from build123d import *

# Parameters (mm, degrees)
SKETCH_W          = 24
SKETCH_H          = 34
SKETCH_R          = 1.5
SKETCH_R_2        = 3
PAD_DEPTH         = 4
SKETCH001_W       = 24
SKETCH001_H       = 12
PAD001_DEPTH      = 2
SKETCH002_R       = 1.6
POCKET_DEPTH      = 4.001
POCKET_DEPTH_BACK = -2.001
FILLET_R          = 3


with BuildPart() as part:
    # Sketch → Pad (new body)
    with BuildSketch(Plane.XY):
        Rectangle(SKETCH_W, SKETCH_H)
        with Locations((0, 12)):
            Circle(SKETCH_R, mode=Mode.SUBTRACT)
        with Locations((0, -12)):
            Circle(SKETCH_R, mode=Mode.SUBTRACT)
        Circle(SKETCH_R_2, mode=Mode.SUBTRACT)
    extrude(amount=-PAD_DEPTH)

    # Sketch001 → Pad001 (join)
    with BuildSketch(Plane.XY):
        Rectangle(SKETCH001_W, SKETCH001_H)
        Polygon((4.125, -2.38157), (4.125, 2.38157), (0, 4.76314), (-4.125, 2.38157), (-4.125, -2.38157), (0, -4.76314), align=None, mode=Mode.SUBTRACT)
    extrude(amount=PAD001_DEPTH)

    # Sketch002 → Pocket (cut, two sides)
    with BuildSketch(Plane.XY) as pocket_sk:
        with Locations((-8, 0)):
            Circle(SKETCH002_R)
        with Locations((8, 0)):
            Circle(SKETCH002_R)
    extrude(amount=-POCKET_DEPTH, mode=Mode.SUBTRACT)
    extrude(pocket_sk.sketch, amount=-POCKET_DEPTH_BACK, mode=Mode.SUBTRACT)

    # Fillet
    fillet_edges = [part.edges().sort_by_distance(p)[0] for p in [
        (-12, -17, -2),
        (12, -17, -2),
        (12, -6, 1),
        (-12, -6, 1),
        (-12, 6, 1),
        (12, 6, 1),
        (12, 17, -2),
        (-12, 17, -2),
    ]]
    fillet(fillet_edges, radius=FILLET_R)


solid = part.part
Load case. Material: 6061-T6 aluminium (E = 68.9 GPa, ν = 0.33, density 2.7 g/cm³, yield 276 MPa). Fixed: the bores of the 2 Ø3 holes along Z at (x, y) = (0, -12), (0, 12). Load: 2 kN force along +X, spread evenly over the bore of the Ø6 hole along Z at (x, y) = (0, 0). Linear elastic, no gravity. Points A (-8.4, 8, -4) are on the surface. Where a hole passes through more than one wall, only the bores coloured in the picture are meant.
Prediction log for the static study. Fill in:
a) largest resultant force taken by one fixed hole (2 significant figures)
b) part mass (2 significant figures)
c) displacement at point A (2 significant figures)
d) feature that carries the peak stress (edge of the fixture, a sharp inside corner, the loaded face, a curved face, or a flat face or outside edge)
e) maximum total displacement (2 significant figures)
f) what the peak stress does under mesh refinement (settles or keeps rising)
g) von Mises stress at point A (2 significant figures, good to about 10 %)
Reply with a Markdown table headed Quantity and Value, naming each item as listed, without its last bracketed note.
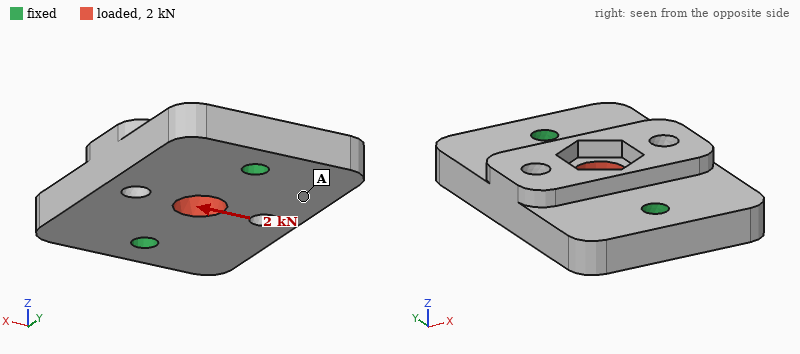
| Quantity | Value |
|---|---|
| largest resultant force taken by one fixed hole | 1.0 kN |
| part mass | 9.2 g |
| displacement at point A | 3.5 µm |
| feature that carries the peak stress | edge of the fixture |
| maximum total displacement | 7.8 µm |
| what the peak stress does under mesh refinement | keeps rising |
| von Mises stress at point A | 14 MPa |
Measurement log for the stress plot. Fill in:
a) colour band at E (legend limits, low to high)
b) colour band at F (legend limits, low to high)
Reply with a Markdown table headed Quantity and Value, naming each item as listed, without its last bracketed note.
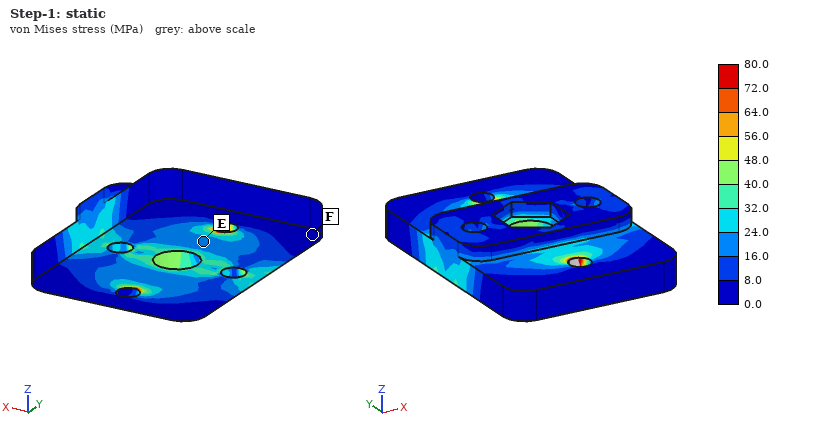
| Quantity | Value |
|---|---|
| colour band at E | 16.0 to 24.0 MPa |
| colour band at F | 0.0 to 8.0 MPa |
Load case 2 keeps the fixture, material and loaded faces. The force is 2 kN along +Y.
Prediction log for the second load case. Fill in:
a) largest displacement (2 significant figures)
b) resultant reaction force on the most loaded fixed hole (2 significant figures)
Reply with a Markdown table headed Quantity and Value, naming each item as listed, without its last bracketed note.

| Quantity | Value |
|---|---|
| largest displacement | 4.3 µm |
| resultant reaction force on the most loaded fixed hole | 1.0 kN |
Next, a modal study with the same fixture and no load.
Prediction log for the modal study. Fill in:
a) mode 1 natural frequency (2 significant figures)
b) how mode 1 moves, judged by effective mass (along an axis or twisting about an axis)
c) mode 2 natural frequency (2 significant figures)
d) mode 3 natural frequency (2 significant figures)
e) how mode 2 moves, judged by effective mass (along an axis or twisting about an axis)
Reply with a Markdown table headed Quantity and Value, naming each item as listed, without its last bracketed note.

| Quantity | Value |
|---|---|
| mode 1 natural frequency | 15 kHz |
| how mode 1 moves, judged by effective mass | twisting about Y |
| mode 2 natural frequency | 20 kHz |
| mode 3 natural frequency | 27 kHz |
| how mode 2 moves, judged by effective mass | along Z |
